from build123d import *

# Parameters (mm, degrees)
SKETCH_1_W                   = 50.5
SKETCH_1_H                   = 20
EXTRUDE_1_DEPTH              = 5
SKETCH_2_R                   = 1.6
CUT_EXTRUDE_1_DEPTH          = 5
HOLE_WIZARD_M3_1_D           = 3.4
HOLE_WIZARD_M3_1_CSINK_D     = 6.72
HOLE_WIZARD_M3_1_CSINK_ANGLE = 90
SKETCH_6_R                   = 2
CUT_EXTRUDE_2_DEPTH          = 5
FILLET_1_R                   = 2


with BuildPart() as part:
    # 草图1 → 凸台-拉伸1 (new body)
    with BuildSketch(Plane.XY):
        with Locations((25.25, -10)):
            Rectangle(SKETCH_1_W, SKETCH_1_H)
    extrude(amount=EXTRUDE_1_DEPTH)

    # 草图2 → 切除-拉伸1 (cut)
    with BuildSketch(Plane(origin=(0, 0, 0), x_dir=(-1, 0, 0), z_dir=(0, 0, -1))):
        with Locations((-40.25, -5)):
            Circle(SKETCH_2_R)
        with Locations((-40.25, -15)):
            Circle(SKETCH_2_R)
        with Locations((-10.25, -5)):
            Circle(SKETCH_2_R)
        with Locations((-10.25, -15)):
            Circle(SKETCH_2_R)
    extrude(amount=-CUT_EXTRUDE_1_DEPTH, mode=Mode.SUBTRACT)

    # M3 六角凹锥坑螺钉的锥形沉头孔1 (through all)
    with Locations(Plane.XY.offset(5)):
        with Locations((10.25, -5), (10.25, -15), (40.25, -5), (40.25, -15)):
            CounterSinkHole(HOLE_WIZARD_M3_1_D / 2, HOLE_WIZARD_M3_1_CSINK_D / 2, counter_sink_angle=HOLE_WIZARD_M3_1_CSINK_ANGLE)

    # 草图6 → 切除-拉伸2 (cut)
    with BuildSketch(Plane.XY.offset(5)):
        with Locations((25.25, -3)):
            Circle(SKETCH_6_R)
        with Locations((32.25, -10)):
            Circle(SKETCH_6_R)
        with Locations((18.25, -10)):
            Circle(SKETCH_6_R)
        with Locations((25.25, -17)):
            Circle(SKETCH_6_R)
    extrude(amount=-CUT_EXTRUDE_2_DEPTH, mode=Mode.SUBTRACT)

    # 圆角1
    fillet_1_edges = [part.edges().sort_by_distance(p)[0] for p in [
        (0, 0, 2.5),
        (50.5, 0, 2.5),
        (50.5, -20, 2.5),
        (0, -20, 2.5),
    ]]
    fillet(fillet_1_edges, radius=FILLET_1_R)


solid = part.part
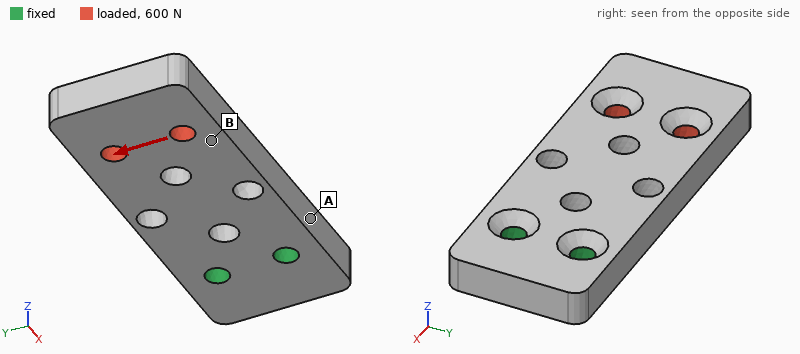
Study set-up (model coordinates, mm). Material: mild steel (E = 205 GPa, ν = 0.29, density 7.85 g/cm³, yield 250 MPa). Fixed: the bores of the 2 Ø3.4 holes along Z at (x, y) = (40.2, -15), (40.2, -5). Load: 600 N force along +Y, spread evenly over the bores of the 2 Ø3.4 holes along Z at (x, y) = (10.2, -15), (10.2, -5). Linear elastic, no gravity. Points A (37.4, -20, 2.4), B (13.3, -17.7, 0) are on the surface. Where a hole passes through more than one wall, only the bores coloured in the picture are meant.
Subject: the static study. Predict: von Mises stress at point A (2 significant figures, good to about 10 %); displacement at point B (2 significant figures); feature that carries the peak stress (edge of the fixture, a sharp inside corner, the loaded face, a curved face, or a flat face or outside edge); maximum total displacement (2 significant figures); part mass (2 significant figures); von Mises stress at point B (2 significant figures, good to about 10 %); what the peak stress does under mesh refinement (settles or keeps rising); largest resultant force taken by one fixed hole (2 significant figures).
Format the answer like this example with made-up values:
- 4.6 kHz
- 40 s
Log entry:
- 43 MPa
- 15 µm
- edge of the fixture
- 23 µm
- 35 g
- 12 MPa
- keeps rising
- 1.5 kN
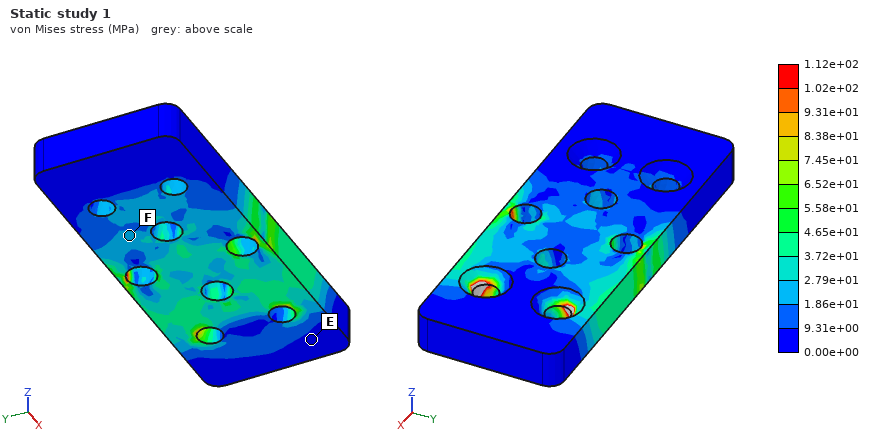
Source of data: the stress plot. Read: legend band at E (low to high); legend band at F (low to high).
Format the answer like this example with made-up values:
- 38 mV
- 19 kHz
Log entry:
- 0.00e+00 to 9.31e+00 MPa
- 1.86e+01 to 2.79e+01 MPa
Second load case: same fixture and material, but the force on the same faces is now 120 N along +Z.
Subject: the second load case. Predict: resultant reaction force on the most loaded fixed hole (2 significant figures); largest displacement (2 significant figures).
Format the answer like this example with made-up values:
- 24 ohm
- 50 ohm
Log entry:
- 62 N
- 52 µm
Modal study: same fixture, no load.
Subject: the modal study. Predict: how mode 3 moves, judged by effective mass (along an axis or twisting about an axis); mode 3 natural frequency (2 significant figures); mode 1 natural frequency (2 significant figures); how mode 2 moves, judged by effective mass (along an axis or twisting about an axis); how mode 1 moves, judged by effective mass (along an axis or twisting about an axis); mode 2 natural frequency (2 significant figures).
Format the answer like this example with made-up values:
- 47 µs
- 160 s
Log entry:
- twisting about X
- 8900 Hz
- 2300 Hz
- along Y
- along Z
- 7500 Hz
